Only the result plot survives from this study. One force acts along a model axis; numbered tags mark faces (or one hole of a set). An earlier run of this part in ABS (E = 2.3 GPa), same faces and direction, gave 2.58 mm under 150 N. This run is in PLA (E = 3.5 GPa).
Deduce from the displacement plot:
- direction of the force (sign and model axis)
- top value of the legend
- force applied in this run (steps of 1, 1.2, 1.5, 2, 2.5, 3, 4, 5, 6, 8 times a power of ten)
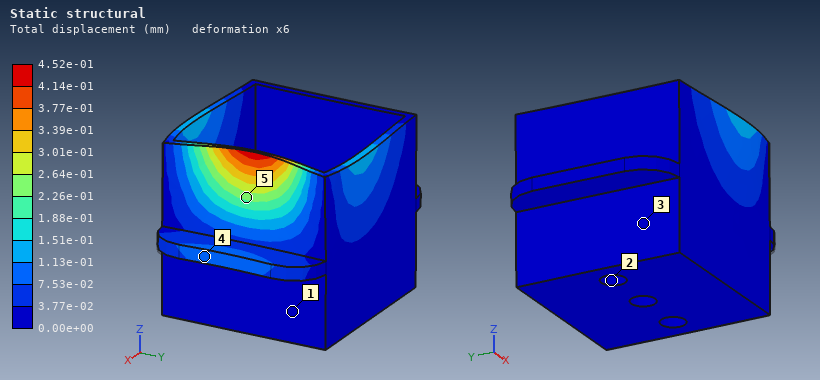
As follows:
-X
4.52e-01 mm
40 N
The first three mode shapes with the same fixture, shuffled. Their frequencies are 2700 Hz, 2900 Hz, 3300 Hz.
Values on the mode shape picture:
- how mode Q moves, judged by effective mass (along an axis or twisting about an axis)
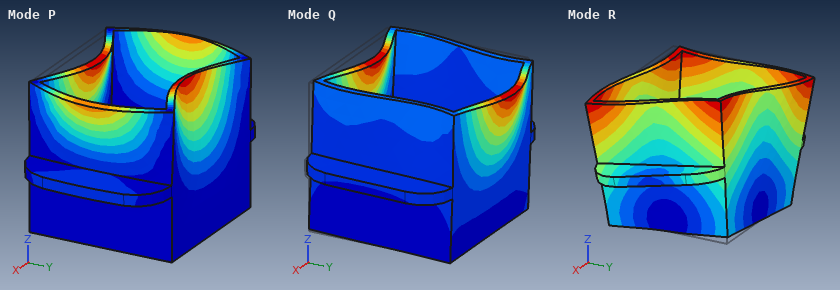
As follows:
along Y
